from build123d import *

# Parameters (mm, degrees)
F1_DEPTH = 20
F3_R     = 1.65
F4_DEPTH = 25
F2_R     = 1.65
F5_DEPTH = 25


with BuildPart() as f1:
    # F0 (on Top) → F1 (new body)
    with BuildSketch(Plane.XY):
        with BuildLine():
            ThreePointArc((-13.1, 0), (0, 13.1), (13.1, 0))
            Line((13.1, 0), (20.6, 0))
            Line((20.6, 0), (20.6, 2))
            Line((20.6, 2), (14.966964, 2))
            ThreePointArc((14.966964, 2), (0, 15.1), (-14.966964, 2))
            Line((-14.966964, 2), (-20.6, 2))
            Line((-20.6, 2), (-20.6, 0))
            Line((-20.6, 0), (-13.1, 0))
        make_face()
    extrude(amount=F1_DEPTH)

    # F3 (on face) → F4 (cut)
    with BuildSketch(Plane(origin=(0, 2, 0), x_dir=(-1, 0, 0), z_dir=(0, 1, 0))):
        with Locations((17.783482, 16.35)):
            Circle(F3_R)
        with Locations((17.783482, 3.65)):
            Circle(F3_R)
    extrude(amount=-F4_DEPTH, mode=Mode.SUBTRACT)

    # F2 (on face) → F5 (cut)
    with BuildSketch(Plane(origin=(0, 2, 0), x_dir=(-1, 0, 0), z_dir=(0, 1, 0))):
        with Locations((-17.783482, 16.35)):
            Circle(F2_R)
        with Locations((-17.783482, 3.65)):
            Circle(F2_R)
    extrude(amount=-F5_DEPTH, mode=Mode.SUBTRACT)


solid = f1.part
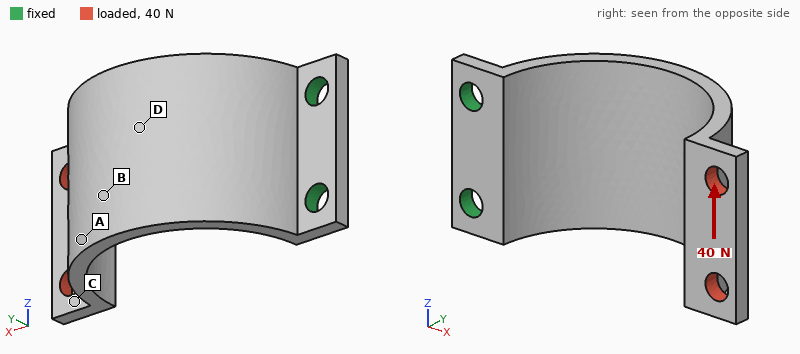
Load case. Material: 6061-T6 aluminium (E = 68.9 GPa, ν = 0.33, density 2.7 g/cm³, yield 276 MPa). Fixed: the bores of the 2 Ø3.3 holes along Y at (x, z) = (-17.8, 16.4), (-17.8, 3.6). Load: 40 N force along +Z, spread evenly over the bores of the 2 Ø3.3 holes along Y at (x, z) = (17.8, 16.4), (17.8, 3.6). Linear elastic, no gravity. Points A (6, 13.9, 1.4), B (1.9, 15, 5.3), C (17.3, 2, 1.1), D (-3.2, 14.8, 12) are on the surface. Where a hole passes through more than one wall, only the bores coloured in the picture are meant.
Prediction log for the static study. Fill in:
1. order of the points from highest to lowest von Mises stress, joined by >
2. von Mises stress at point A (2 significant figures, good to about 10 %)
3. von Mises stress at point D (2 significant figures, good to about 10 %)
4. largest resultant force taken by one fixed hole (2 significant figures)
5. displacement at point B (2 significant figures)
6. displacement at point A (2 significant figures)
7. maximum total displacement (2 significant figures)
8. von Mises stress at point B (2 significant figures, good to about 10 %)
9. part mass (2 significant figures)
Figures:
D > B > A > C
20 MPa
42 MPa
97 N
0.081 mm
0.15 mm
0.37 mm
29 MPa
5.8 g
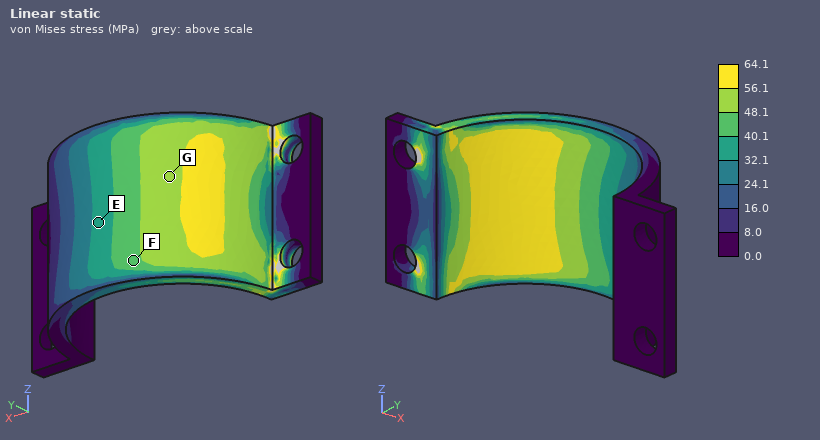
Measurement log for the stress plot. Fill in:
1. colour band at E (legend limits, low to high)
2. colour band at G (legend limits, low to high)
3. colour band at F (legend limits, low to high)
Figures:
32.1 to 40.1 MPa
48.1 to 56.1 MPa
40.1 to 48.1 MPa
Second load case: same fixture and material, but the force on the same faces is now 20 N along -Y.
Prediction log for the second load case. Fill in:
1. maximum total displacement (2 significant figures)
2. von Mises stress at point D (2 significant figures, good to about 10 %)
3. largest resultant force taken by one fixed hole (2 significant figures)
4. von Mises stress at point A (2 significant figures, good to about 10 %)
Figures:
0.48 mm
26 MPa
11 N
18 MPa
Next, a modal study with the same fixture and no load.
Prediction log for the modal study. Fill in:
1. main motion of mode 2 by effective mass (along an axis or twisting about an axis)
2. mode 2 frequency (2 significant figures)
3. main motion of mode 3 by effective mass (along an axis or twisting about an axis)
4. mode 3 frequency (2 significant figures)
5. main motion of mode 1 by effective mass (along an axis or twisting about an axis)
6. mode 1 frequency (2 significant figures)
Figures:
along Z
1400 Hz
along X
2600 Hz
along Y
830 Hz
